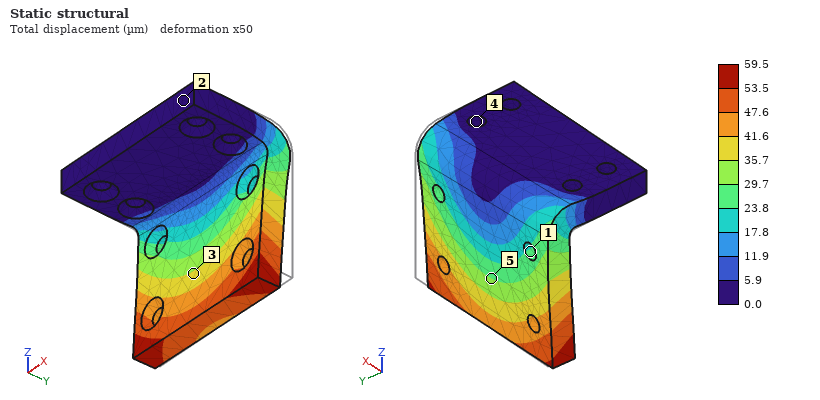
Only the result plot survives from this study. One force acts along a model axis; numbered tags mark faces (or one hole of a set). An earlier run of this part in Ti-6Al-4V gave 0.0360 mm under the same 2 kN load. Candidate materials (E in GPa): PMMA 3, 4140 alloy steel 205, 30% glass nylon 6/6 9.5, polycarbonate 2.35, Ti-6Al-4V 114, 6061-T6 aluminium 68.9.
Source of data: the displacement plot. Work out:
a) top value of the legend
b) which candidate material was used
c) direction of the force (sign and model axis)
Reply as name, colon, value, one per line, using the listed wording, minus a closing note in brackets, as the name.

top value of the legend: 59.5 µm
which candidate material was used: 6061-T6 aluminium
direction of the force: -X
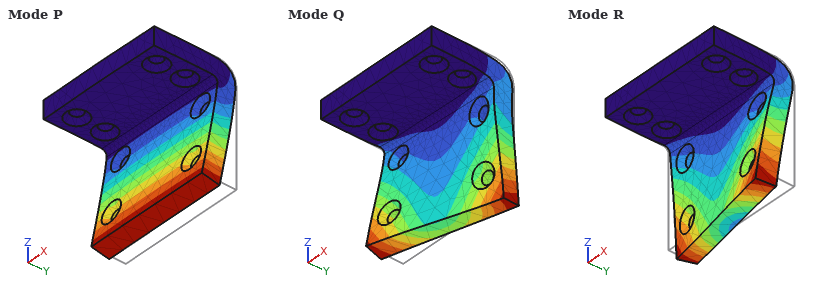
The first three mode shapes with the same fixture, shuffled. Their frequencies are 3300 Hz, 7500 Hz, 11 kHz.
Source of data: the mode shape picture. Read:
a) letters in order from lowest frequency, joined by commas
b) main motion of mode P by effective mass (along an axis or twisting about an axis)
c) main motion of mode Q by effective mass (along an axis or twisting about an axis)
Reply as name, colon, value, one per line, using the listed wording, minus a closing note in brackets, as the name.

letters in order from lowest frequency, joined by commas: P, R, Q
main motion of mode P by effective mass: along Y
main motion of mode Q by effective mass: along X
